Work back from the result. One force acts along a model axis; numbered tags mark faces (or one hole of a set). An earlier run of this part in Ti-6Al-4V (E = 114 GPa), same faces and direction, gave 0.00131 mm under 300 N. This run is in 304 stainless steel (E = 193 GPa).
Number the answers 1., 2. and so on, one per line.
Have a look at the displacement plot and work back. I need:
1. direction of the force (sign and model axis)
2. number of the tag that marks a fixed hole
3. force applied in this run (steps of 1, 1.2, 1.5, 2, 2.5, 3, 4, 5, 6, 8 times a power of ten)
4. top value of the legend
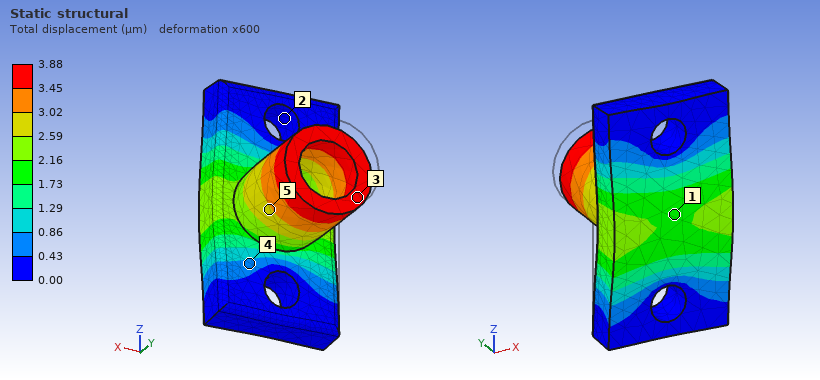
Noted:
1. -Y
2. 2
3. 1.5 kN
4. 3.88 µm
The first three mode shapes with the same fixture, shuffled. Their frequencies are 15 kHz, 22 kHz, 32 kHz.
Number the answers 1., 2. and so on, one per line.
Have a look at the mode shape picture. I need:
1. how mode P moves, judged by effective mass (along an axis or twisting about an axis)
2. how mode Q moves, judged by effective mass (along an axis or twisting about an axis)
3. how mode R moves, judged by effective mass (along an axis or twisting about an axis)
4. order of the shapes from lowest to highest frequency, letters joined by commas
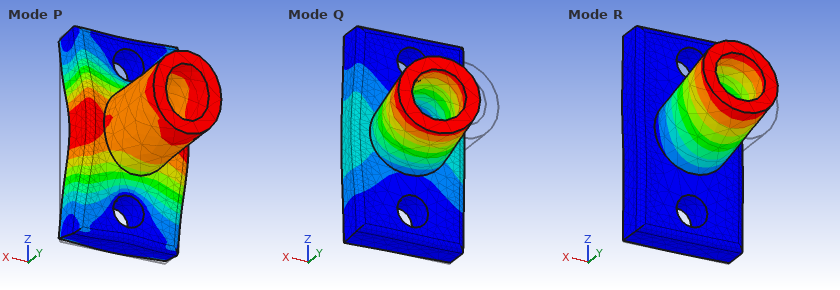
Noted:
1. along Y
2. along X
3. along Z
4. Q, R, P
